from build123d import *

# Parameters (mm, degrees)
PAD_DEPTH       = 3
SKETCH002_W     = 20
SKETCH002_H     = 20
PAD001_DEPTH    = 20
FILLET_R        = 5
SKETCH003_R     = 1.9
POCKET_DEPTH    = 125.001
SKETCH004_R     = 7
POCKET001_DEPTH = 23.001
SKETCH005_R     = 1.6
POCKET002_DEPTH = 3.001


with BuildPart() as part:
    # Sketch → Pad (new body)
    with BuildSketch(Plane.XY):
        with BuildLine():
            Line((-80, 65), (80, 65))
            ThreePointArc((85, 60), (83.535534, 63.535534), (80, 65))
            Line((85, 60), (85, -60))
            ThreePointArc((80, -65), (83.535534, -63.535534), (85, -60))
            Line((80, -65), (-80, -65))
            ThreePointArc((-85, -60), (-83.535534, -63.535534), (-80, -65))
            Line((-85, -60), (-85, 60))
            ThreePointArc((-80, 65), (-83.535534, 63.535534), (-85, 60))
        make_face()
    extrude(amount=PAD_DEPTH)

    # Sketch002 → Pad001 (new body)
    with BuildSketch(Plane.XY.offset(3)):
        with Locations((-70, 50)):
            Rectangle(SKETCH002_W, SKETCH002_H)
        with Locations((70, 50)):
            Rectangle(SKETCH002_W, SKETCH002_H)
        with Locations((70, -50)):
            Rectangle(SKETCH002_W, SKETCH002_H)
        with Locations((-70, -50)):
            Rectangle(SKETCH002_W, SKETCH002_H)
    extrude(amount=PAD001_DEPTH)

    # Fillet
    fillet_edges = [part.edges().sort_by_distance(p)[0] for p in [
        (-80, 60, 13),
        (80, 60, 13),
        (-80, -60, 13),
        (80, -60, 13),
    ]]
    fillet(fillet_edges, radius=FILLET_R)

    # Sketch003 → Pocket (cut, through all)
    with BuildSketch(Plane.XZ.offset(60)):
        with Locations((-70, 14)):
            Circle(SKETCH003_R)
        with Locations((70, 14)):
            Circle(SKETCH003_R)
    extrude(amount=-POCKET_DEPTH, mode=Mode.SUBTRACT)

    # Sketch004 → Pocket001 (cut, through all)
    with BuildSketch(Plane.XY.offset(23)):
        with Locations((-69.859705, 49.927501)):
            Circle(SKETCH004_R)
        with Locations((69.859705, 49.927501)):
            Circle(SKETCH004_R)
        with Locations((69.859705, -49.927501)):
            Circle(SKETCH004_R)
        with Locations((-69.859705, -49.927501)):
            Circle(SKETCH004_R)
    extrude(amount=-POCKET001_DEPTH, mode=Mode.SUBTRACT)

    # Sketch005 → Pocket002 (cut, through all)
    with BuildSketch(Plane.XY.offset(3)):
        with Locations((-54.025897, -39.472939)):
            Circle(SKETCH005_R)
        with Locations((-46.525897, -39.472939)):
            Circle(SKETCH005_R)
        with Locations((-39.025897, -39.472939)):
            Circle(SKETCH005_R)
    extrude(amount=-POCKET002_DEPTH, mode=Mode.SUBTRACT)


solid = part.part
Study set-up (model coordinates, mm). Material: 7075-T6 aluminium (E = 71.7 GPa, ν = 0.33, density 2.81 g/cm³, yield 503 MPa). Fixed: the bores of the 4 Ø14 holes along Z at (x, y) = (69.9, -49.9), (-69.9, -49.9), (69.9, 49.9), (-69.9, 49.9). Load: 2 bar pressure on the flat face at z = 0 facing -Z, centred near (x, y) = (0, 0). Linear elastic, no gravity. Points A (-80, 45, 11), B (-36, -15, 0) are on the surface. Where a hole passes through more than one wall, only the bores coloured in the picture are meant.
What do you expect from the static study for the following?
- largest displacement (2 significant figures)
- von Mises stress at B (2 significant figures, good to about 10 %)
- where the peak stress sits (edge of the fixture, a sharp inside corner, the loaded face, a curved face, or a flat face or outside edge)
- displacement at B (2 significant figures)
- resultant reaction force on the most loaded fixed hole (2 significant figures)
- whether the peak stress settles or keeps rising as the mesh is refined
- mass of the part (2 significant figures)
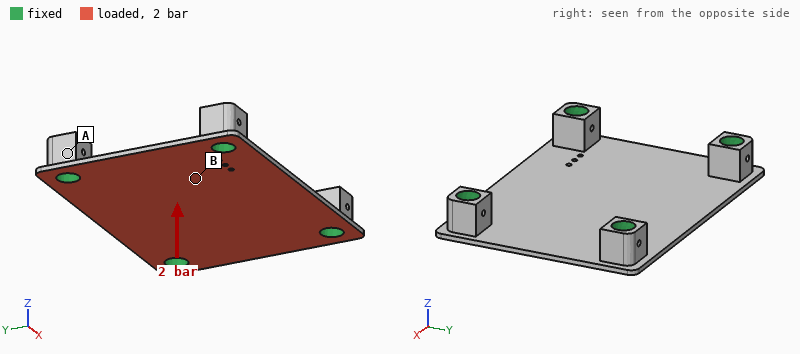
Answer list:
1.1 mm
43 MPa
a sharp inside corner
0.67 mm
1.1 kN
keeps rising
230 g
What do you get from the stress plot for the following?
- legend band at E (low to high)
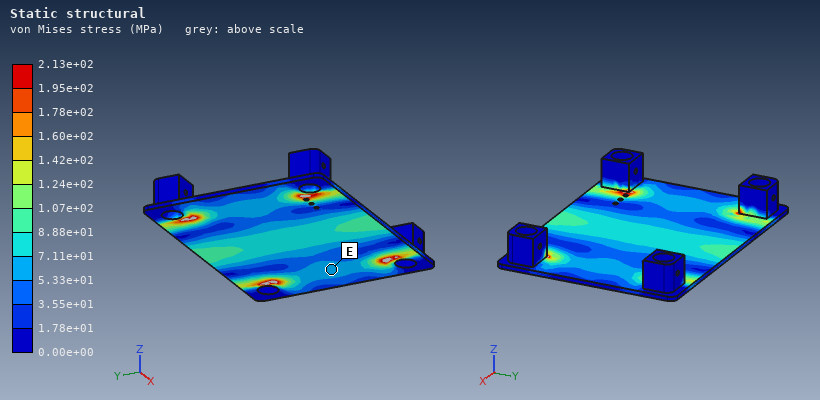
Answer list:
5.33e+01 to 7.11e+01 MPa
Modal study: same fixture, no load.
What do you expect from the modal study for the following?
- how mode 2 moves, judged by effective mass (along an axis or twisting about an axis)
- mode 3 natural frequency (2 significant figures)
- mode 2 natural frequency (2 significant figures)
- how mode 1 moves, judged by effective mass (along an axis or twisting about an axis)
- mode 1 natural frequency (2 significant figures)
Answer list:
twisting about X
1700 Hz
1200 Hz
along Z
880 Hz
